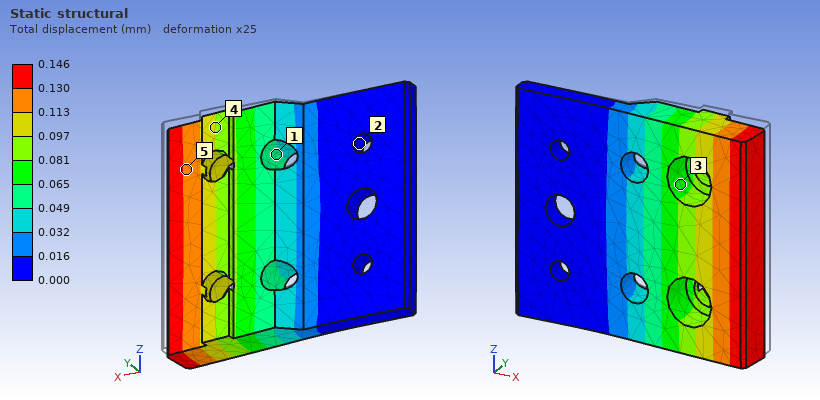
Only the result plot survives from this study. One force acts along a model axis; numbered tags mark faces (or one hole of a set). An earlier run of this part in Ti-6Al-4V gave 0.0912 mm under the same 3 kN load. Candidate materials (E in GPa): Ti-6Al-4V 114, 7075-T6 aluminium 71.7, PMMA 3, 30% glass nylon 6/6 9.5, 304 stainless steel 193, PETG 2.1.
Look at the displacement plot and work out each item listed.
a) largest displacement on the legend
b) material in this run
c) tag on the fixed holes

0.146 mm
7075-T6 aluminium
2
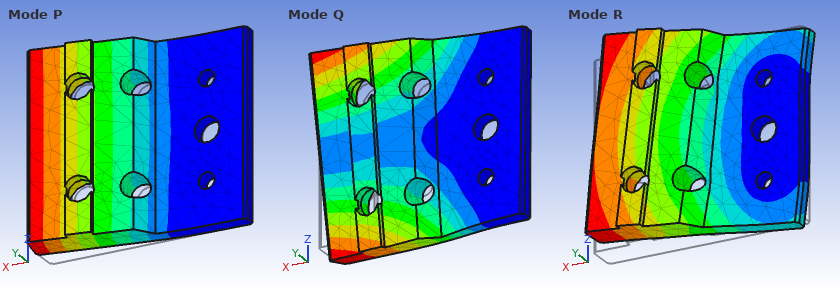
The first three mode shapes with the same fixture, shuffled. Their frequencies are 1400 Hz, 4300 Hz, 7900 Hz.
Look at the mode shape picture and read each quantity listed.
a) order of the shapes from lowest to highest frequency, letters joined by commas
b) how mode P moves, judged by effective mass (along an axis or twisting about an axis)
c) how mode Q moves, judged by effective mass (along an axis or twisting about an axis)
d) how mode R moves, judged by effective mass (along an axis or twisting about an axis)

P, Q, R
along Y
twisting about X
along Z
